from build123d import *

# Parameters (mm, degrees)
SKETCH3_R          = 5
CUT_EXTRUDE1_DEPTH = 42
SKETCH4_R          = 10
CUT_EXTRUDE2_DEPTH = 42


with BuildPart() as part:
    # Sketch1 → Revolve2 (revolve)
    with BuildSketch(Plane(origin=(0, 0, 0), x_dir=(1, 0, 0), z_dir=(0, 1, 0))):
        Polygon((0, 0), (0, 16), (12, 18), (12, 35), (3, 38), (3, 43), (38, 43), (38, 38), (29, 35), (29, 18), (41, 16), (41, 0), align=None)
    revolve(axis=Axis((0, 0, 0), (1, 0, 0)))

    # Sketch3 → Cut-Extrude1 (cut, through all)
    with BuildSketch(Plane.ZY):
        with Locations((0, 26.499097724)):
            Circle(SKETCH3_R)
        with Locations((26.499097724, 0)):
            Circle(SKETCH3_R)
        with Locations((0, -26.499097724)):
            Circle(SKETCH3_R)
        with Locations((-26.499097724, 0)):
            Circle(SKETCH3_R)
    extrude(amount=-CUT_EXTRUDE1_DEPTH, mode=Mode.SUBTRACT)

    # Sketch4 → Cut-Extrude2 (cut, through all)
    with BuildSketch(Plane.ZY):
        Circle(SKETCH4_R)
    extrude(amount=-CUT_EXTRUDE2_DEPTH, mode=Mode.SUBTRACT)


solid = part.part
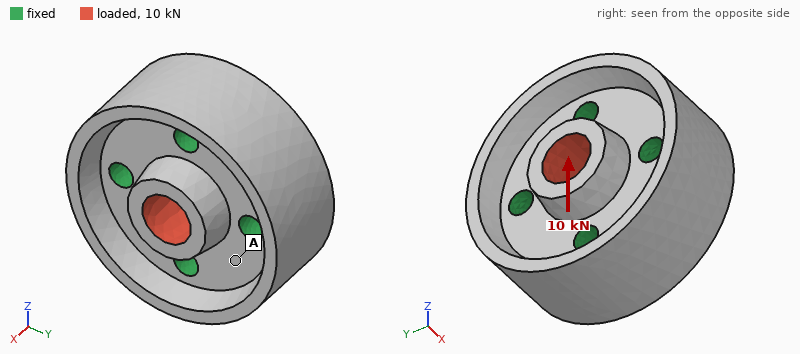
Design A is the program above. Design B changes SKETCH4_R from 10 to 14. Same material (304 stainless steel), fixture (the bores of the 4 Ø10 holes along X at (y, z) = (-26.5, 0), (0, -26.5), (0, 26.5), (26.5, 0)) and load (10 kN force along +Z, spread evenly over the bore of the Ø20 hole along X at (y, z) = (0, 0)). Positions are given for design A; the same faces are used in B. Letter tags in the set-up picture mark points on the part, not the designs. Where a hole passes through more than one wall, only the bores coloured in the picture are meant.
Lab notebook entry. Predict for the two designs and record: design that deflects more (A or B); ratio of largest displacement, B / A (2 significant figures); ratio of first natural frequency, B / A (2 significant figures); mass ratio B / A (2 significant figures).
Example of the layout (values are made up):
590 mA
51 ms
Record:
B
2.1
0.98
0.91
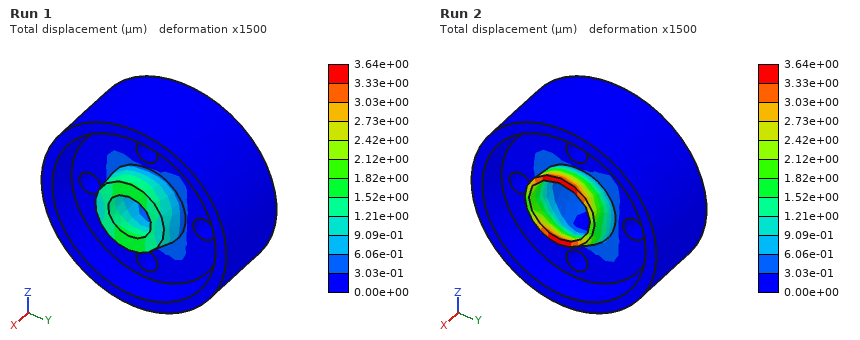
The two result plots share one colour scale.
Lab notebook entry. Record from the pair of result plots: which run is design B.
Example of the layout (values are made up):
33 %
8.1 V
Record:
Run 2
